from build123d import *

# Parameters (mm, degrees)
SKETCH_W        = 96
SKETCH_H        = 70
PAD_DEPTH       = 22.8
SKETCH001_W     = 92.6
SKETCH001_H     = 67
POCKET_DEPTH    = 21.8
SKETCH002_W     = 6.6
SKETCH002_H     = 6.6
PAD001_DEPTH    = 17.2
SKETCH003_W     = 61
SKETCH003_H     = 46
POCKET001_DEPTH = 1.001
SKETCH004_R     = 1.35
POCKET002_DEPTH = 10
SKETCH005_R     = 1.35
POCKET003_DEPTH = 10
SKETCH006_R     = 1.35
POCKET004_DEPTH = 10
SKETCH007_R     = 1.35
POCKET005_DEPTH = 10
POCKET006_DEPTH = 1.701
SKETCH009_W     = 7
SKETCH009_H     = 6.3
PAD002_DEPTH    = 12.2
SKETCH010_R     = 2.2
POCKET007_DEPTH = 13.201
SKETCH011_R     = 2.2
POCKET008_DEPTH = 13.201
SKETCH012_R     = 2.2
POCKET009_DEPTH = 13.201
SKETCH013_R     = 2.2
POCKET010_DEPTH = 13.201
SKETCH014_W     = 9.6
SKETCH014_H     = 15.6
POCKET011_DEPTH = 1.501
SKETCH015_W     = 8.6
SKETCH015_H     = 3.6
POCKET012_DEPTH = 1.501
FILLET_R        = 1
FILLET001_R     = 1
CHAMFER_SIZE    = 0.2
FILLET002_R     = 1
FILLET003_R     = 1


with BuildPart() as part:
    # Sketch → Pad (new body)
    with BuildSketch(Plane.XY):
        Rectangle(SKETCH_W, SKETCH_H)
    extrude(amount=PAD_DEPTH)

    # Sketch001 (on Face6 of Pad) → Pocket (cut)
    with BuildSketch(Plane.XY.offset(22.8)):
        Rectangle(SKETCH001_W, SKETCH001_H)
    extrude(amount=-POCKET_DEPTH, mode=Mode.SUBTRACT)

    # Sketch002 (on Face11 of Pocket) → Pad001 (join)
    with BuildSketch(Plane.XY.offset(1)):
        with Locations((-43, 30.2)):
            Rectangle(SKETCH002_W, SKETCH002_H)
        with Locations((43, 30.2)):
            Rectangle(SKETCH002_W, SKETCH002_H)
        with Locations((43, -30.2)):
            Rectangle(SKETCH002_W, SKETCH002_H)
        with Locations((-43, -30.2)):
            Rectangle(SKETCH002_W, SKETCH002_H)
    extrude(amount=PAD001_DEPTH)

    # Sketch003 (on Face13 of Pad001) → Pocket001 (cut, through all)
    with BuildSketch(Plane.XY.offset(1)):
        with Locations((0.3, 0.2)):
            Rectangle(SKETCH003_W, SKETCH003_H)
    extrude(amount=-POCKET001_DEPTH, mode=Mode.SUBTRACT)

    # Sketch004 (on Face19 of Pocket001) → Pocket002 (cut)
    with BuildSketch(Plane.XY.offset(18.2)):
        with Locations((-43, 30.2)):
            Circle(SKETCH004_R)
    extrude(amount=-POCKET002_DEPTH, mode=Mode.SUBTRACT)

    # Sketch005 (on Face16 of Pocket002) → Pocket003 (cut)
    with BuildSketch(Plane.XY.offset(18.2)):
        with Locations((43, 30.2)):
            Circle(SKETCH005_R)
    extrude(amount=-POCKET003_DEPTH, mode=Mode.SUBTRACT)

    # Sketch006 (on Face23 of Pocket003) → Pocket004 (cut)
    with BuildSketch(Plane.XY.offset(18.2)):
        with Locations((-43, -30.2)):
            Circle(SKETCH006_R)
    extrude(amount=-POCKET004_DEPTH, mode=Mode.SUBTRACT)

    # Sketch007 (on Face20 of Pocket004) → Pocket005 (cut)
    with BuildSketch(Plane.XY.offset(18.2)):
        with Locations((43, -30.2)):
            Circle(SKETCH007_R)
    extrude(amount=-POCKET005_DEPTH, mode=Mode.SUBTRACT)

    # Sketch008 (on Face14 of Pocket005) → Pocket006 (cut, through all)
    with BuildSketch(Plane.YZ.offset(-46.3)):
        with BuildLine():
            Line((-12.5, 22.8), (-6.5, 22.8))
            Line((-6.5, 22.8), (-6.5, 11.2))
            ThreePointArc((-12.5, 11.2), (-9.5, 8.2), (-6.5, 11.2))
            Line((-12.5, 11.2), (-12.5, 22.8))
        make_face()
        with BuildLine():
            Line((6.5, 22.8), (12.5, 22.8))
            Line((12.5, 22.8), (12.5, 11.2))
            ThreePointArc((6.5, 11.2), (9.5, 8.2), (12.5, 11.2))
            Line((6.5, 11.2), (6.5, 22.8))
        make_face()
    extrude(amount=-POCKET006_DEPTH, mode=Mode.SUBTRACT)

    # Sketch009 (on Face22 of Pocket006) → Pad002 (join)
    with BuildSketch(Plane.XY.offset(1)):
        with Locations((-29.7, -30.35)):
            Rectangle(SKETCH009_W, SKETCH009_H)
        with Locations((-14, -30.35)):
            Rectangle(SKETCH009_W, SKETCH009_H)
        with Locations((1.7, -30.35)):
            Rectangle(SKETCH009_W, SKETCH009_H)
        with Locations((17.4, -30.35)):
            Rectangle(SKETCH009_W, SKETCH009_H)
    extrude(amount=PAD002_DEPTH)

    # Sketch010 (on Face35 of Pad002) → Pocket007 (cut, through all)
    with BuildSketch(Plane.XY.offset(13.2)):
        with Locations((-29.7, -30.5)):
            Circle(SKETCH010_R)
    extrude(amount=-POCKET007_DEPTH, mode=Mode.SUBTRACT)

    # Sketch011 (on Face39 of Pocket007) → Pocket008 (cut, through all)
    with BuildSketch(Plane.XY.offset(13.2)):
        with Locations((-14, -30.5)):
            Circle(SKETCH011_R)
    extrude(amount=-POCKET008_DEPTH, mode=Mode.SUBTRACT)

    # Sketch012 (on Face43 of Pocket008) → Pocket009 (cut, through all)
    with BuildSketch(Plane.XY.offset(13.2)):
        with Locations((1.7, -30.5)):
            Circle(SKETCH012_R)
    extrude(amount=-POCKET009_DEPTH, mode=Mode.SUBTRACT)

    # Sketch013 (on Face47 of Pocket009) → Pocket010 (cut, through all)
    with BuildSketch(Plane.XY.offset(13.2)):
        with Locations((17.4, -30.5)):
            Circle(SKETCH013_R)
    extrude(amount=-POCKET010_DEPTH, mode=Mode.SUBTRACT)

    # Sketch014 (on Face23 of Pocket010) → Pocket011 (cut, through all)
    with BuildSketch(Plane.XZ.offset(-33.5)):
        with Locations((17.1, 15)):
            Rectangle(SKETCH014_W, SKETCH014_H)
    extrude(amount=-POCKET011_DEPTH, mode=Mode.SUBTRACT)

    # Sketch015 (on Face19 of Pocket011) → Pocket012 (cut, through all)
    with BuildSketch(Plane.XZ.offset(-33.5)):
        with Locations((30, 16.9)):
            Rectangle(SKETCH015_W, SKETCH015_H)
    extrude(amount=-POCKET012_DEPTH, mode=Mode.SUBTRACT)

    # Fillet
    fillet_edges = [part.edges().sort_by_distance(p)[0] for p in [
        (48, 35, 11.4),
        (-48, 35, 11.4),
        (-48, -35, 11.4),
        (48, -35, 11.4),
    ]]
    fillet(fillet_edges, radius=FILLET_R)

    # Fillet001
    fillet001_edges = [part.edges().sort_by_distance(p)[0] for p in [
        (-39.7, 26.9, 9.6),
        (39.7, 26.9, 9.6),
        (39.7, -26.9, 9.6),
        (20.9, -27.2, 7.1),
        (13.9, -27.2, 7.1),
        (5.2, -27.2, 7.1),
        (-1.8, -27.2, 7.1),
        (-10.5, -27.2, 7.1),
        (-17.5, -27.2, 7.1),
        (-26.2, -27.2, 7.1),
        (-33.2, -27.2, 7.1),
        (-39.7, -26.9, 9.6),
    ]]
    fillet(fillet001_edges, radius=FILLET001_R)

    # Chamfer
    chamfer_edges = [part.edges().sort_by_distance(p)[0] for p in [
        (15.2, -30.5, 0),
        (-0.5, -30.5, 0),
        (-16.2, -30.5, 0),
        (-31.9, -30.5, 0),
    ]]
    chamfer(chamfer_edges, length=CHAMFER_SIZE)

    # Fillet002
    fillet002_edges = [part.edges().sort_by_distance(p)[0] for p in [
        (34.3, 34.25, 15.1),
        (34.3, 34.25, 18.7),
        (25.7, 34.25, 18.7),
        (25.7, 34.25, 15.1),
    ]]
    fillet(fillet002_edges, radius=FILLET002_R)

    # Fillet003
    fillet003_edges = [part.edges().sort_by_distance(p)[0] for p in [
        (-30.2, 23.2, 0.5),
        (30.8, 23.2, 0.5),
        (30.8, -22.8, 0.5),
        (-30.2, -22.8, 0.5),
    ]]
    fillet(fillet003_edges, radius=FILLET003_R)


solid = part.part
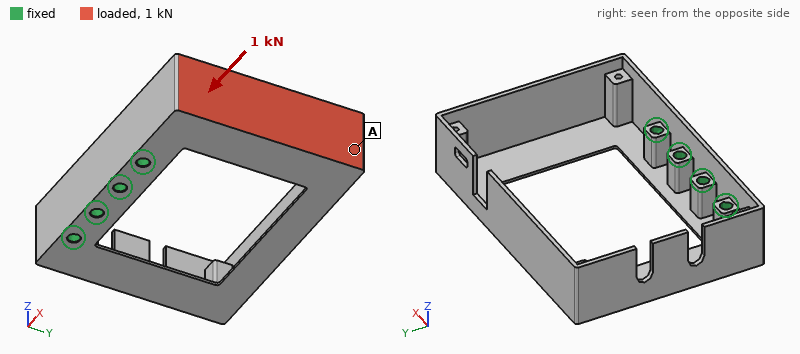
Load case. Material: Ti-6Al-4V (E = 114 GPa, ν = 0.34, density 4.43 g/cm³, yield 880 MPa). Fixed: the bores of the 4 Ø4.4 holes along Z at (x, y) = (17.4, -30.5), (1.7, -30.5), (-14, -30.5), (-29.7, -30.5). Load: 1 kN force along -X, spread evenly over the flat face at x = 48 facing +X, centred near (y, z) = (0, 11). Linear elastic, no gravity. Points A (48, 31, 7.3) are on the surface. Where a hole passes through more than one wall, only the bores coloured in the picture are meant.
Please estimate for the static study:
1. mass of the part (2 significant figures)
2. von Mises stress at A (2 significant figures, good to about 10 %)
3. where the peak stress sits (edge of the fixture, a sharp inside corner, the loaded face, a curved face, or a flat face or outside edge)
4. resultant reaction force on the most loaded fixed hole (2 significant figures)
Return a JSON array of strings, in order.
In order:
["83 g", "36 MPa", "a curved face", "500 N"]
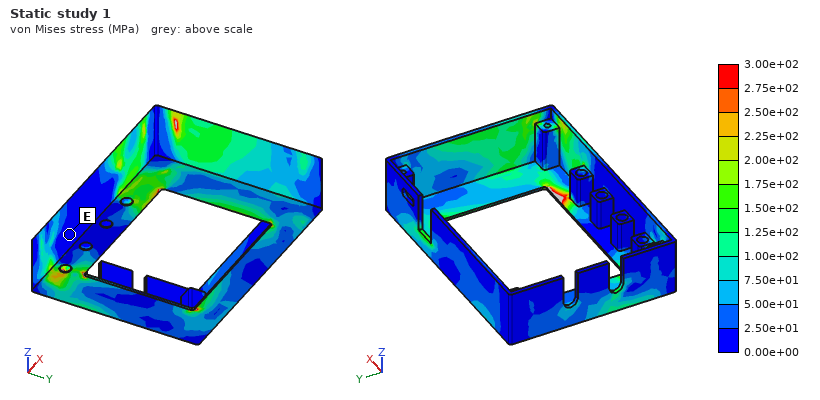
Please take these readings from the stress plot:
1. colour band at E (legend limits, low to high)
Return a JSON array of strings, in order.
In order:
["0.00e+00 to 2.50e+01 MPa"]
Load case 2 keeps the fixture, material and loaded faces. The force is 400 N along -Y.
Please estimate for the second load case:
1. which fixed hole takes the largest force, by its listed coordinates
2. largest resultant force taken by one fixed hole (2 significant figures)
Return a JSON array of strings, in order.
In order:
["(17.4, -30.5)", "550 N"]
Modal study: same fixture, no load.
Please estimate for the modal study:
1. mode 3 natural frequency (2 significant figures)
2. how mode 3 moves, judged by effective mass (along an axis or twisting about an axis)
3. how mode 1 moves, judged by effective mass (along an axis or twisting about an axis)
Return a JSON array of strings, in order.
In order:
["1100 Hz", "along X", "along Z"]
